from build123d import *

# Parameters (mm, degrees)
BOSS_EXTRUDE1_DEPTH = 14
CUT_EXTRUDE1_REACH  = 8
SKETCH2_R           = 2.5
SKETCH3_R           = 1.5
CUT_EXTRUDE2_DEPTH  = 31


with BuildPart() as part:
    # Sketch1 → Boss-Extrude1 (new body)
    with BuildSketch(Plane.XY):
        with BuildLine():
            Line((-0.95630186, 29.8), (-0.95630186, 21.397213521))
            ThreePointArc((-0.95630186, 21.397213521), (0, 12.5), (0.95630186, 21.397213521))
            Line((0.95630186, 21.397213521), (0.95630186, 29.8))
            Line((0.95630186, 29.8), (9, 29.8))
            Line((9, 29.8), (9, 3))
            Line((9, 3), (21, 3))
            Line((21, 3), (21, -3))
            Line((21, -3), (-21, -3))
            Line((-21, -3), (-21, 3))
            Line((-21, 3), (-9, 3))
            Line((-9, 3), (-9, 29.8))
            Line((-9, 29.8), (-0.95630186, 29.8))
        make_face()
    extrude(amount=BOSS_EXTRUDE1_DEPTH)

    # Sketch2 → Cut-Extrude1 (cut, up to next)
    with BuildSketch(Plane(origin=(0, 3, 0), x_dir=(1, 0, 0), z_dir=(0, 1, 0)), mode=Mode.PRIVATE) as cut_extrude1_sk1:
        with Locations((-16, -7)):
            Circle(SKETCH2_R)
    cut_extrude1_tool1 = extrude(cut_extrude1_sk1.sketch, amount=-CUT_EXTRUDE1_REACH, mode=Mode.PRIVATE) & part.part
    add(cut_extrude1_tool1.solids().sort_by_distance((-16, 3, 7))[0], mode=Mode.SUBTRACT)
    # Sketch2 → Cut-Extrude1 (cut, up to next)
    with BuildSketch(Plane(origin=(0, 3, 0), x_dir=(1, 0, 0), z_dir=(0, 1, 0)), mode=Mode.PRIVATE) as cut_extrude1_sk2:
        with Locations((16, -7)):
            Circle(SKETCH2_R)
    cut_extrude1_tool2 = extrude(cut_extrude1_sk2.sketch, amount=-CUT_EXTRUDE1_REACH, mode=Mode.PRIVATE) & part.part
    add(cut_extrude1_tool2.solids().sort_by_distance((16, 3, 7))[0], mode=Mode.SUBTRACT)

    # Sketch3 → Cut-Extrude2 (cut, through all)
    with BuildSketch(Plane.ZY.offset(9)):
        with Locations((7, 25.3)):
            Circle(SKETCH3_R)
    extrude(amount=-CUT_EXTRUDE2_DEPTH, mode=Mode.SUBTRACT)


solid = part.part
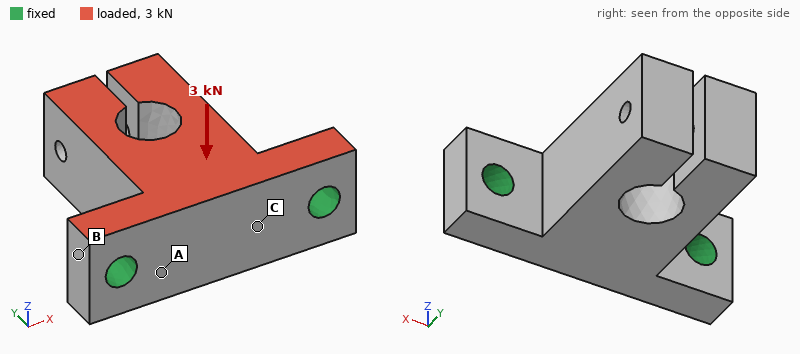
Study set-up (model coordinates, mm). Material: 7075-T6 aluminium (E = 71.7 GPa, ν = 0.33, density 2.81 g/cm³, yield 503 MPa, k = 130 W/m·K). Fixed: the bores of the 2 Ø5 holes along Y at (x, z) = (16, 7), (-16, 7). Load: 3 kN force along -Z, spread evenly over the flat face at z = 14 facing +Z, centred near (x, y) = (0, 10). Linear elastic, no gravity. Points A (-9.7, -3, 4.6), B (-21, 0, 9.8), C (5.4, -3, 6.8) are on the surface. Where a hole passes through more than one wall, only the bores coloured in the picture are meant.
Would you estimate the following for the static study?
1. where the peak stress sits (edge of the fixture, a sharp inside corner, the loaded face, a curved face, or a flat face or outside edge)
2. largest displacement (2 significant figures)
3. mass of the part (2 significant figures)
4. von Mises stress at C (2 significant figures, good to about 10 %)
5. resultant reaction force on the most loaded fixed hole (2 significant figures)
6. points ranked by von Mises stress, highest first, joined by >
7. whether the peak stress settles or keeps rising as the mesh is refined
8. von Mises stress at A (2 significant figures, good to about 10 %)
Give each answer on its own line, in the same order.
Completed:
edge of the fixture
0.18 mm
25 g
38 MPa
1.5 kN
A > C > B
keeps rising
73 MPa
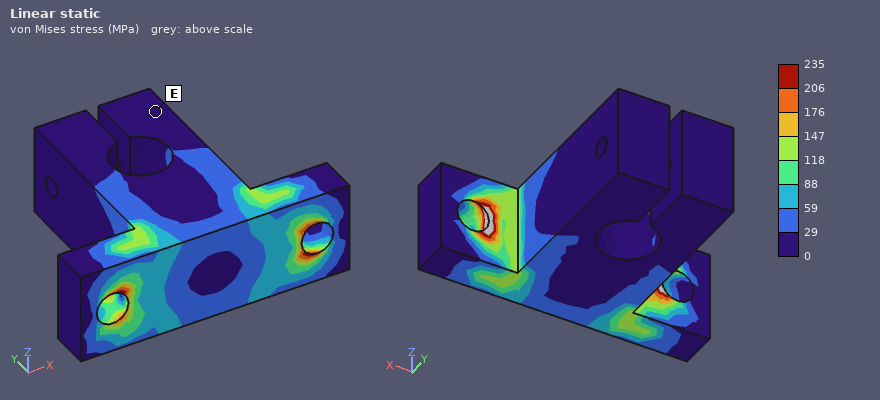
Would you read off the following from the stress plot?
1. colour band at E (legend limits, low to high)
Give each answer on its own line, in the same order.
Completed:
0 to 29 MPa
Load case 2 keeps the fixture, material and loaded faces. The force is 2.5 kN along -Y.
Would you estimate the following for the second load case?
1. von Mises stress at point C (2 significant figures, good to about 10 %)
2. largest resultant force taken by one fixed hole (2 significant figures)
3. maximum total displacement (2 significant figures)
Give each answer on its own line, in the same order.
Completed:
31 MPa
1.3 kN
88 µm
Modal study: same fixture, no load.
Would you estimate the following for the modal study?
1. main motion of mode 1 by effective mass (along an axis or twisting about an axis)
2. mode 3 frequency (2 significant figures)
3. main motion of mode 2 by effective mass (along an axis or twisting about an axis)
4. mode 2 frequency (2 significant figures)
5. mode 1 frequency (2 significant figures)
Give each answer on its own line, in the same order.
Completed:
along Z
8800 Hz
along X
7600 Hz
5000 Hz
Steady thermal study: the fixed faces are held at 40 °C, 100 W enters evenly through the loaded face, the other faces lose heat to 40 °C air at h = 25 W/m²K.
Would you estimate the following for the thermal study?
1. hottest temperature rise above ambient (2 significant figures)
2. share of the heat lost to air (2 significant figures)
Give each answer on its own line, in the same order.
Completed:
70 K
3.4 %
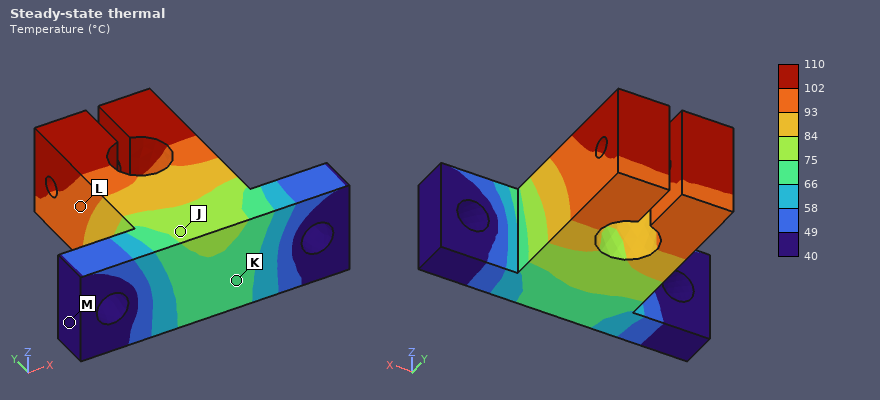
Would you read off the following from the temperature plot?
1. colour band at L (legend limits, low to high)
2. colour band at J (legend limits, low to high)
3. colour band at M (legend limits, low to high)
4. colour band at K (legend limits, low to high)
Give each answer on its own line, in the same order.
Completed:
93 to 102 °C
75 to 84 °C
40 to 49 °C
66 to 75 °C
